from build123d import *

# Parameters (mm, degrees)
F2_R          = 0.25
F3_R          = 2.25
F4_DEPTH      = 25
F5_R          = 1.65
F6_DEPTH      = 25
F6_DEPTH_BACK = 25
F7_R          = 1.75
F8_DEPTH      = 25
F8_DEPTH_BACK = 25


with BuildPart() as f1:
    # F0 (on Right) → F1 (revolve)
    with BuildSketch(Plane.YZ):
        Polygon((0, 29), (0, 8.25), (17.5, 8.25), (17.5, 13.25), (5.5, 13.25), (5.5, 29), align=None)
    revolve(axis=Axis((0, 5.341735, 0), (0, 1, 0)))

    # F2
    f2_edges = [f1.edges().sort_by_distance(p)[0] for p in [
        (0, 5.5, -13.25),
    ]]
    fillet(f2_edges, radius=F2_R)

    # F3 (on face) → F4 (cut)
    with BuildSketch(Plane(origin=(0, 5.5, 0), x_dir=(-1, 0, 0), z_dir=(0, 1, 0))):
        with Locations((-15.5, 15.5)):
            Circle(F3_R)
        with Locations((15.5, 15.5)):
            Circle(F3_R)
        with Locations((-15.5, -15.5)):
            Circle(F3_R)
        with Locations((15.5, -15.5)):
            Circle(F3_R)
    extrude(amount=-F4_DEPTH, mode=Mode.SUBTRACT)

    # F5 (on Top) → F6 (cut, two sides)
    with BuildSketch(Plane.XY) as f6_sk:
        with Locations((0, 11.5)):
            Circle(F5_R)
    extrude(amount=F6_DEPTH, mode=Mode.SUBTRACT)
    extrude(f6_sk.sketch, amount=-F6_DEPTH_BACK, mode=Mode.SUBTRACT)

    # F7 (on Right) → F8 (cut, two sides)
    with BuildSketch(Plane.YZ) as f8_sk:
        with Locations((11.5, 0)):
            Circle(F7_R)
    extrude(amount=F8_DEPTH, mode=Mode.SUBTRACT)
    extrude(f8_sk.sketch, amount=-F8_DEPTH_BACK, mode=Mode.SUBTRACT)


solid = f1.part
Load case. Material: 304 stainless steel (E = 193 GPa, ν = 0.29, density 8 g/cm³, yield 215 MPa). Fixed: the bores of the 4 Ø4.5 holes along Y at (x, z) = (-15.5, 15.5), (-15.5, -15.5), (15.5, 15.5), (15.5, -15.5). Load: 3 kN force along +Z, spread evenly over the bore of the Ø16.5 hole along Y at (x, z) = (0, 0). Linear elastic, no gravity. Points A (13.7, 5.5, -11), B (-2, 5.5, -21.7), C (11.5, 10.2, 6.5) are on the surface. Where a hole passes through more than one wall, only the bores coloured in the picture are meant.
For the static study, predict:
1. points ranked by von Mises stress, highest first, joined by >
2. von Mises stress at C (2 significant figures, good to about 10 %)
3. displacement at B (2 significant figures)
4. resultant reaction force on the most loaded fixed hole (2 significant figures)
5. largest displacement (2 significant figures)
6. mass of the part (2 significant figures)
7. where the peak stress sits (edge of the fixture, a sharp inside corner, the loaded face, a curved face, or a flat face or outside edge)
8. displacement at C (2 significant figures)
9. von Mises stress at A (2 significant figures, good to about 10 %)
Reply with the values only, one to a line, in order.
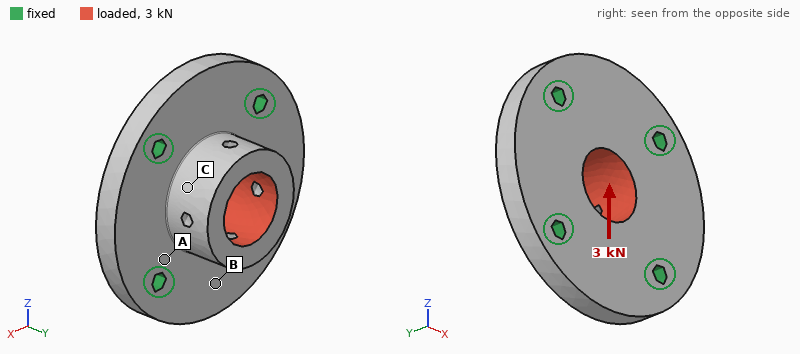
A > C > B
7.4 MPa
1.1 µm
830 N
3.8 µm
140 g
a curved face
1.9 µm
16 MPa
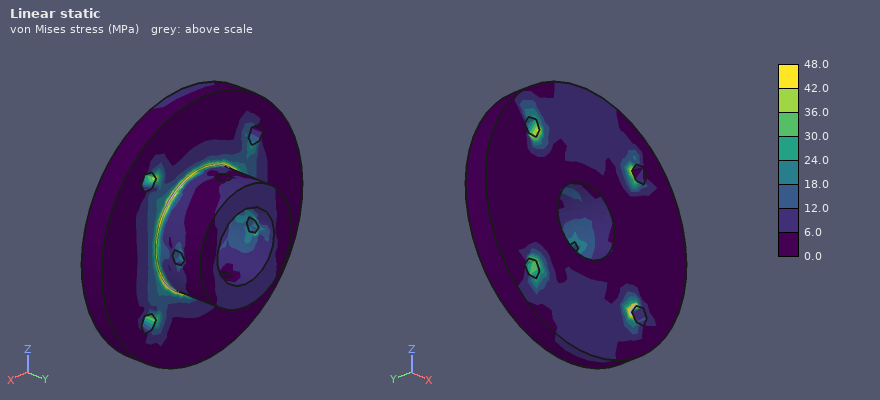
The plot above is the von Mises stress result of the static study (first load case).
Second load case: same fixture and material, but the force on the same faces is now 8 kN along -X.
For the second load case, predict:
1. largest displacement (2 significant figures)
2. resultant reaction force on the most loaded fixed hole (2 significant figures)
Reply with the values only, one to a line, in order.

10 µm
2.2 kN
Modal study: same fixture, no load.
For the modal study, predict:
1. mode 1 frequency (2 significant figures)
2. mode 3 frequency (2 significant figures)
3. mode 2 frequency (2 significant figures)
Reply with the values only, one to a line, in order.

19 kHz
19 kHz
19 kHz
